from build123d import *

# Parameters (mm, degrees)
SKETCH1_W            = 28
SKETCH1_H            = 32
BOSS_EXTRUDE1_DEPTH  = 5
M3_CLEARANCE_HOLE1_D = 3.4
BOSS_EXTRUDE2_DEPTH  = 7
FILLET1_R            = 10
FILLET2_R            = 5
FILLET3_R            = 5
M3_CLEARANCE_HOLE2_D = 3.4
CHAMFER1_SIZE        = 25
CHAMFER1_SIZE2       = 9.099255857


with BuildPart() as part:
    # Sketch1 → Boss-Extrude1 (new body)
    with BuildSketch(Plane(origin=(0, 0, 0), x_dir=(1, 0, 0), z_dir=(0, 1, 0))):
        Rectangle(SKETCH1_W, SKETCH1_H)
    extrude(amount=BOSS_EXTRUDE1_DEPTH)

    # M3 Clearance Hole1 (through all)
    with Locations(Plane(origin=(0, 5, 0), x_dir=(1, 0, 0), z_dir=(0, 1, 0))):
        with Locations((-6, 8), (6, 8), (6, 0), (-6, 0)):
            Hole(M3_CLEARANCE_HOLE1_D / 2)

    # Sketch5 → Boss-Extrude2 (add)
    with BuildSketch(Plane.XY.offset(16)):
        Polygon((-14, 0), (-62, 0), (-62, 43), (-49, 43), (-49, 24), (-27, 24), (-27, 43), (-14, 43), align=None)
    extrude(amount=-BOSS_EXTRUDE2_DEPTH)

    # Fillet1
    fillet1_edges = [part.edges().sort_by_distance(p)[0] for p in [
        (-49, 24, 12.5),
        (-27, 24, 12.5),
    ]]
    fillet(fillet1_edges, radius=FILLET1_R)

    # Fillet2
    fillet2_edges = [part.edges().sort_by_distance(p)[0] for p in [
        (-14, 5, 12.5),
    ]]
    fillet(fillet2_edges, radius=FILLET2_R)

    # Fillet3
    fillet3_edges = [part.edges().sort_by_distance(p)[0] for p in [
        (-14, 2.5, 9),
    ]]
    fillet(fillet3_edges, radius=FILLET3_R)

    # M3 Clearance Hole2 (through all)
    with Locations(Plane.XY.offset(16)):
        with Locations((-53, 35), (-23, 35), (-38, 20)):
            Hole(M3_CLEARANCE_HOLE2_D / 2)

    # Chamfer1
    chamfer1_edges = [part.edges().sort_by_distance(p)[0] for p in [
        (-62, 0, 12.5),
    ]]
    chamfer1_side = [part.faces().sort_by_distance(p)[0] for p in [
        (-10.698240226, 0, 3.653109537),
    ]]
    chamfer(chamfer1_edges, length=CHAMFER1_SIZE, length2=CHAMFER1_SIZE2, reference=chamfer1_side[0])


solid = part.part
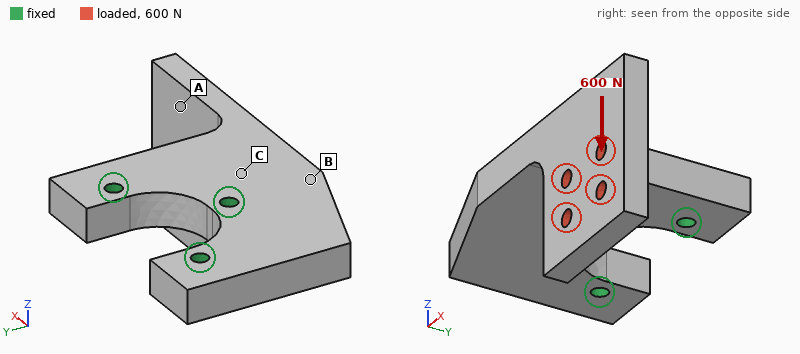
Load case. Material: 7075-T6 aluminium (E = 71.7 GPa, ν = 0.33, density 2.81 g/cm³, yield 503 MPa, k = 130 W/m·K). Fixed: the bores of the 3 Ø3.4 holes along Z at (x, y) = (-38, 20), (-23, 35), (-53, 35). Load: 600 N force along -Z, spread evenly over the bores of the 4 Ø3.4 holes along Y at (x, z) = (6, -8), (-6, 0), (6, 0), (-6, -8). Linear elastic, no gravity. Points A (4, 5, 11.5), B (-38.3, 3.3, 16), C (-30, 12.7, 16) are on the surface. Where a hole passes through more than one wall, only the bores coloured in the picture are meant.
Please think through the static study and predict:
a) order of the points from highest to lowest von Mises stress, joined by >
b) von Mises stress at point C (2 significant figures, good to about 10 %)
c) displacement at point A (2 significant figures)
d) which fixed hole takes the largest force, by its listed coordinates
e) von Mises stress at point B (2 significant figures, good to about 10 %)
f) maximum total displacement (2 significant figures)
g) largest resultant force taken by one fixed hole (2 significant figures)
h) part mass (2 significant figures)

C > B > A
68 MPa
0.35 mm
(-38, 20)
46 MPa
0.60 mm
460 N
43 g
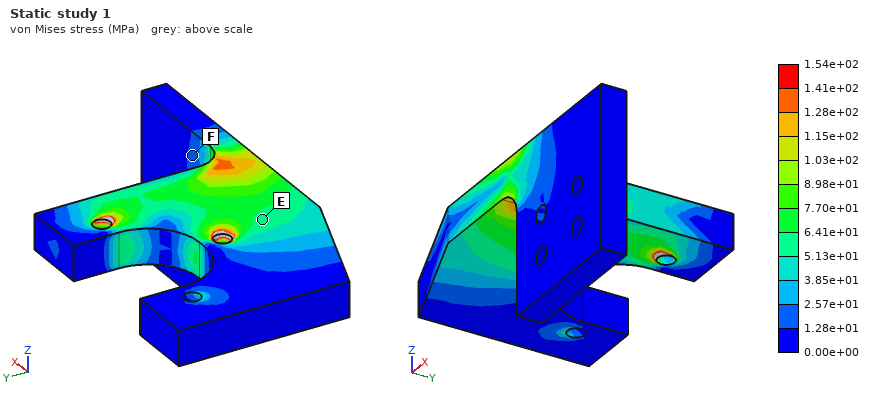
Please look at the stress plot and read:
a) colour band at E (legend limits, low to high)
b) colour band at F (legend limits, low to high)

5.13e+01 to 6.41e+01 MPa
1.28e+01 to 2.57e+01 MPa
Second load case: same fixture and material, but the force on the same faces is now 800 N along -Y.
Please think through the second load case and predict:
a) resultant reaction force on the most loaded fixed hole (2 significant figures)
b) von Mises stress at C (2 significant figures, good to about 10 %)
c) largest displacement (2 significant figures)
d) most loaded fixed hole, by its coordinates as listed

1.3 kN
51 MPa
0.91 mm
(-23, 35)
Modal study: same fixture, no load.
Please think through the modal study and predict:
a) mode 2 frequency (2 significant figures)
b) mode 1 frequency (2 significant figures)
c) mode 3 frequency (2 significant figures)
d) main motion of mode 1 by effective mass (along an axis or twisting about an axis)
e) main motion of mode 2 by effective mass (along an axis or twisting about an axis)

2100 Hz
1600 Hz
4300 Hz
along Z
along Y
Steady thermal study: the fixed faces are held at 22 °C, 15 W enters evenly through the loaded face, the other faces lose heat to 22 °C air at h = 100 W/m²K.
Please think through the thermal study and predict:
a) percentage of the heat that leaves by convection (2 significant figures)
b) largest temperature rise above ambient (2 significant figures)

49 %
33 K
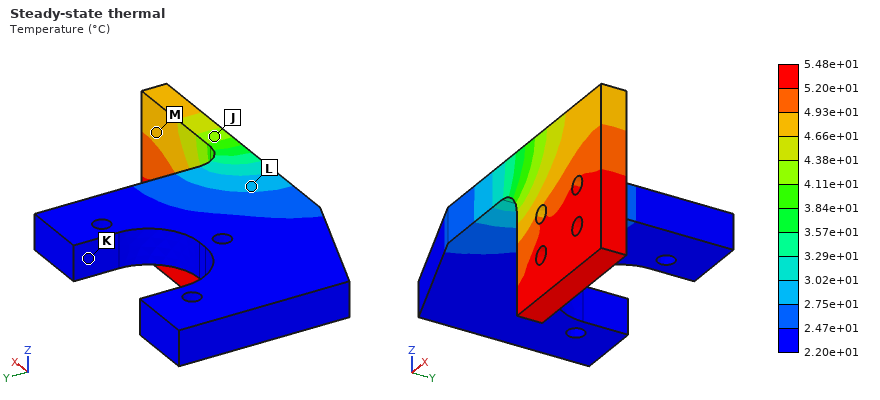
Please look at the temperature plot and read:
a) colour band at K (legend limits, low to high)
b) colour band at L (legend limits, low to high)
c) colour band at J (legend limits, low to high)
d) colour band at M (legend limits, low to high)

2.20e+01 to 2.47e+01 °C
2.75e+01 to 3.02e+01 °C
4.11e+01 to 4.38e+01 °C
4.66e+01 to 4.93e+01 °C
